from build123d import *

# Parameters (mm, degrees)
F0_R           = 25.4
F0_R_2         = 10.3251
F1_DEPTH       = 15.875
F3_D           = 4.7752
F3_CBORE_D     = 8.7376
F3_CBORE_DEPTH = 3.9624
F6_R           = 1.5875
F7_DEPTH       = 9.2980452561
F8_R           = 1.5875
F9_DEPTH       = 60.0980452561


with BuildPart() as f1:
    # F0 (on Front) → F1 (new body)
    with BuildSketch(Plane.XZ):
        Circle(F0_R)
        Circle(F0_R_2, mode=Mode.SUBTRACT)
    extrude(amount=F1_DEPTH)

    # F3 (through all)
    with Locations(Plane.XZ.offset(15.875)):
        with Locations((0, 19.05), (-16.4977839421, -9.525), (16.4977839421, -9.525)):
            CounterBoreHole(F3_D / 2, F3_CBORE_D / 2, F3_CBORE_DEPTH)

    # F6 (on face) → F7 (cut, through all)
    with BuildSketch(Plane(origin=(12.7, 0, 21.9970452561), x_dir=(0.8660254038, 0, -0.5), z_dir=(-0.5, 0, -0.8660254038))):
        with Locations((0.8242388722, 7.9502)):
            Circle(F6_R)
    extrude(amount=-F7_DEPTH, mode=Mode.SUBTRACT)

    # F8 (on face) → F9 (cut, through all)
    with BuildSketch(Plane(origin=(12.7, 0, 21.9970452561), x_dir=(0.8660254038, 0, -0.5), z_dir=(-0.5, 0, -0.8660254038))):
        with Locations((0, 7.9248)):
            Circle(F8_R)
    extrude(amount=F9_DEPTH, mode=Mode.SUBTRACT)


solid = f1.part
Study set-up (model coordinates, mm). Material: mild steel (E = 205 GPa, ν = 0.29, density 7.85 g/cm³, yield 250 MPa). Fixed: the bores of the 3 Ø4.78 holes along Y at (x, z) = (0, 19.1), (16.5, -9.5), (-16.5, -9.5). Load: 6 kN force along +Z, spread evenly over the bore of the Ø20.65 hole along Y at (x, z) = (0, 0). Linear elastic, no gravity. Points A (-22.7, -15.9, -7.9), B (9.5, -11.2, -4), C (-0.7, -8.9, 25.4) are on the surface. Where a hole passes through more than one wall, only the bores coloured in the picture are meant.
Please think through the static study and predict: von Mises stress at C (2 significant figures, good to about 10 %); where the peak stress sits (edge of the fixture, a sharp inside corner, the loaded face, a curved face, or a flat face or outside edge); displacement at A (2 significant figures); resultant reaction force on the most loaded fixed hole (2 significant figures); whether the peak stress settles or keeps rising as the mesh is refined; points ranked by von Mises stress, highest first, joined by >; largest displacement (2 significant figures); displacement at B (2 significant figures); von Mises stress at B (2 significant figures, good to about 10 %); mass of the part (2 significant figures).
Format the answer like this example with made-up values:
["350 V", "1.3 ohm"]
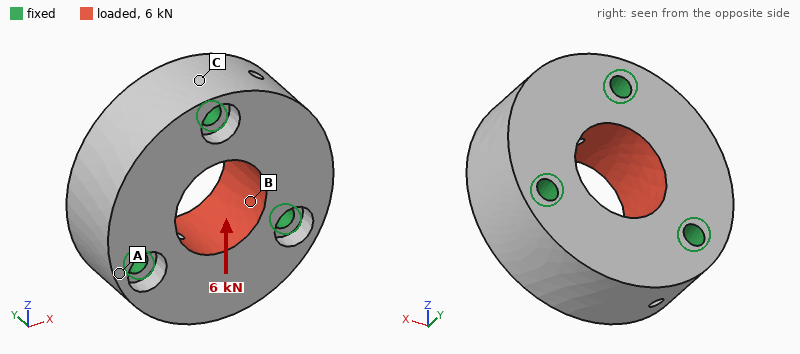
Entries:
["6.1 MPa", "edge of the fixture", "0.26 µm", "2.2 kN", "keeps rising", "B > C > A", "1.4 µm", "0.84 µm", "12 MPa", "200 g"]
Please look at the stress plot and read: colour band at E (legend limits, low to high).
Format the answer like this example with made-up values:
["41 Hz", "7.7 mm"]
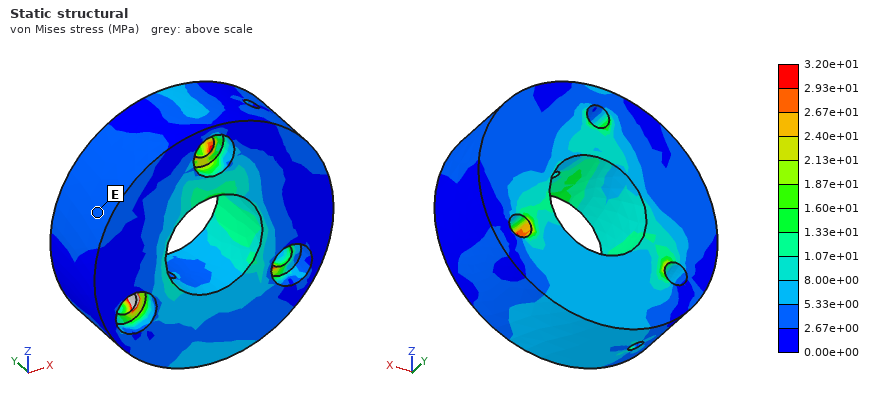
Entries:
["2.67e+00 to 5.33e+00 MPa"]
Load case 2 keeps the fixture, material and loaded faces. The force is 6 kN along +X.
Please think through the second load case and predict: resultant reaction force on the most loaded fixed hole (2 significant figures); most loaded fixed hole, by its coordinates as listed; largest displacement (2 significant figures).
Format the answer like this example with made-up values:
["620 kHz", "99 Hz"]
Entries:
["2.3 kN", "(0, 19.1)", "1.2 µm"]
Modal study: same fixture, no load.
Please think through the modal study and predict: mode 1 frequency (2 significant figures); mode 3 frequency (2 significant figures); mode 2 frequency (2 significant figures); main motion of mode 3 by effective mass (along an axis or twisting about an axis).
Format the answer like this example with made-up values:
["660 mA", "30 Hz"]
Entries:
["22 kHz", "27 kHz", "22 kHz", "along Y"]
